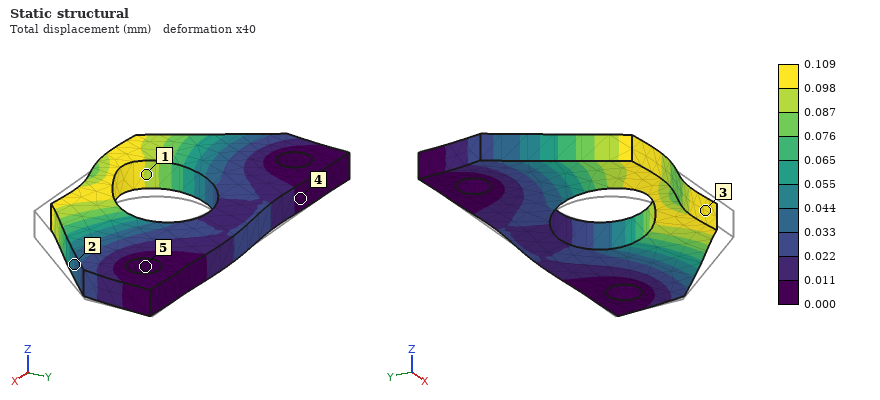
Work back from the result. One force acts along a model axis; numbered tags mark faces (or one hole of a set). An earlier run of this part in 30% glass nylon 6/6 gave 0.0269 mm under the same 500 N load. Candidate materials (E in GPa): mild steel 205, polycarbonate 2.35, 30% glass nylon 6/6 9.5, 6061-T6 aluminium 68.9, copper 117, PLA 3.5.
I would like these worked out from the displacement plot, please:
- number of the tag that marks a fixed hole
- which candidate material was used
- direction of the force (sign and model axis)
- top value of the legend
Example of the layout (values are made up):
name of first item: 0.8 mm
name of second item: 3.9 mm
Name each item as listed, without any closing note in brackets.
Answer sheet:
number of the tag that marks a fixed hole: 5
which candidate material was used: polycarbonate
direction of the force: -X
top value of the legend: 0.109 mm
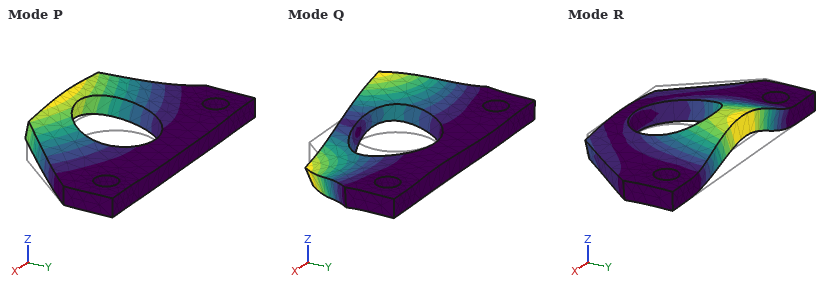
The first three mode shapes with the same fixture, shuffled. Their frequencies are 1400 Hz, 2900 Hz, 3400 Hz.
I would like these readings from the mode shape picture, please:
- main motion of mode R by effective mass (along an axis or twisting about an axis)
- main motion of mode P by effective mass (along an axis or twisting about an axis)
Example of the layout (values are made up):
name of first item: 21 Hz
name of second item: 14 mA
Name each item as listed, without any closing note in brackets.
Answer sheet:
main motion of mode R by effective mass: along Z
main motion of mode P by effective mass: along Z
